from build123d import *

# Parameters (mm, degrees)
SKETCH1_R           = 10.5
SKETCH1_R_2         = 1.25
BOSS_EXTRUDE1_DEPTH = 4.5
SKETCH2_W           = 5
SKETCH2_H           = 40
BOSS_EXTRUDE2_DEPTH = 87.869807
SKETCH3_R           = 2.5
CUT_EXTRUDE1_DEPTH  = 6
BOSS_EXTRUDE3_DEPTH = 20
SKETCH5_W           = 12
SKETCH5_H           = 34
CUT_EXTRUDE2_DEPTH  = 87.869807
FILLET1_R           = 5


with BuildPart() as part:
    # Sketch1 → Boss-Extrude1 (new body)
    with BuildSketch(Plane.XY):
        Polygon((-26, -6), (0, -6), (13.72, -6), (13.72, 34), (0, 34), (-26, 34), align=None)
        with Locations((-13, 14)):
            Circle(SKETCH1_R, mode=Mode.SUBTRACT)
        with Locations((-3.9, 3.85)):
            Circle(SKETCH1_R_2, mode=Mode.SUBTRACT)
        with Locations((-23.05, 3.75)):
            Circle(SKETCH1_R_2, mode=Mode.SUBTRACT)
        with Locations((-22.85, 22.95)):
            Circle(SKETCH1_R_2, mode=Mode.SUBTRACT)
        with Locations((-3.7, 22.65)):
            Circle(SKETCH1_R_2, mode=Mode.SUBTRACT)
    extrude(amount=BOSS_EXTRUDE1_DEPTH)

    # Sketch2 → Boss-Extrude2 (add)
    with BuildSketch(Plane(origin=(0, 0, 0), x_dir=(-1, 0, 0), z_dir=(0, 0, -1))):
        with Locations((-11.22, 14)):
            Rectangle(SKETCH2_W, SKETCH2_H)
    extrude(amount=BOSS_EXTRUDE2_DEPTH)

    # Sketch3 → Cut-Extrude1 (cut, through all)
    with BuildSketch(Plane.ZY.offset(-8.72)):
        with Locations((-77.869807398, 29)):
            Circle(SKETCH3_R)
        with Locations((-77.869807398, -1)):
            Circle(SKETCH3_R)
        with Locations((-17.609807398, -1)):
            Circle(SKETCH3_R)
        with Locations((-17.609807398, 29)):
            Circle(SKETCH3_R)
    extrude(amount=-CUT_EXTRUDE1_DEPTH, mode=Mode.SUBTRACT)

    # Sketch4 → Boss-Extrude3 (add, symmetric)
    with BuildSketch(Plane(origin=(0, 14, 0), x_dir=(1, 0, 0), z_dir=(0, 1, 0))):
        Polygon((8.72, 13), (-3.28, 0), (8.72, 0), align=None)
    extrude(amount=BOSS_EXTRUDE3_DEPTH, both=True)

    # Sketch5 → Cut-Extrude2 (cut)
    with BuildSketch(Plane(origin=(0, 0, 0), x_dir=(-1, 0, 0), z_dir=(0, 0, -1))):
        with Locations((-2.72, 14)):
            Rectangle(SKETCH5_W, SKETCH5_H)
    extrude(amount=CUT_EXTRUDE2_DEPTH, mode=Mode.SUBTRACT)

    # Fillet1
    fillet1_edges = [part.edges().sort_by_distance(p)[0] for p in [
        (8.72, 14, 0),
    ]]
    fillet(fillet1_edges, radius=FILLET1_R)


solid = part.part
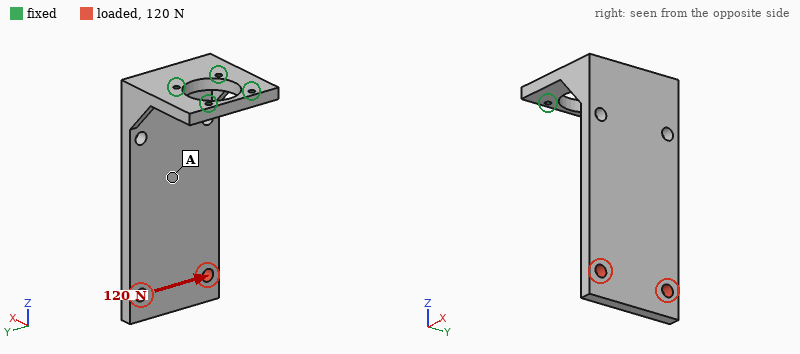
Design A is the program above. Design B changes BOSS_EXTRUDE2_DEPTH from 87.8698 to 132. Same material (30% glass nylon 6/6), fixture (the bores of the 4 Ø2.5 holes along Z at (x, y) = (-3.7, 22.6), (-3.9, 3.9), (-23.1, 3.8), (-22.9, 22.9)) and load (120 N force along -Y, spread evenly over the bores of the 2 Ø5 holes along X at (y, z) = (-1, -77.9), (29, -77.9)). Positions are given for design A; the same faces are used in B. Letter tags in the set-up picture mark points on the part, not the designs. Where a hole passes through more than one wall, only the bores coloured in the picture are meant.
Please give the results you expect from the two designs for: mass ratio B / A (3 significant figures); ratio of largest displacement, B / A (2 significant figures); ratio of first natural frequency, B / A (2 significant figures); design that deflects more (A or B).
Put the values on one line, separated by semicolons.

1.38; 0.89; 0.47; A
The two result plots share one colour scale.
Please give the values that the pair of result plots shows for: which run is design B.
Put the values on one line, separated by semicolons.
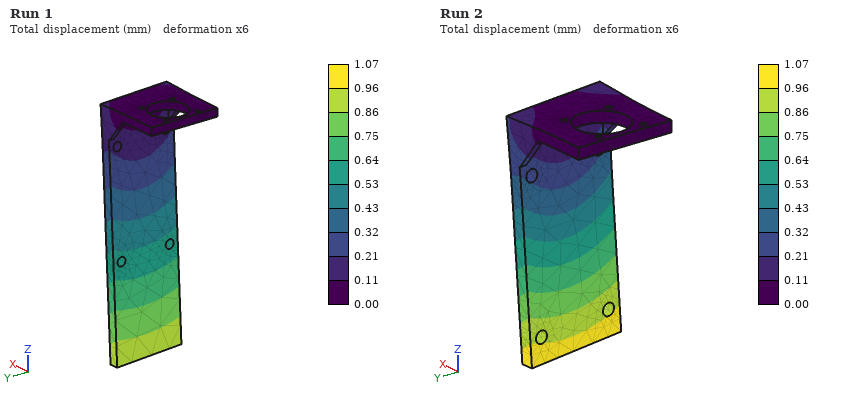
Run 1
